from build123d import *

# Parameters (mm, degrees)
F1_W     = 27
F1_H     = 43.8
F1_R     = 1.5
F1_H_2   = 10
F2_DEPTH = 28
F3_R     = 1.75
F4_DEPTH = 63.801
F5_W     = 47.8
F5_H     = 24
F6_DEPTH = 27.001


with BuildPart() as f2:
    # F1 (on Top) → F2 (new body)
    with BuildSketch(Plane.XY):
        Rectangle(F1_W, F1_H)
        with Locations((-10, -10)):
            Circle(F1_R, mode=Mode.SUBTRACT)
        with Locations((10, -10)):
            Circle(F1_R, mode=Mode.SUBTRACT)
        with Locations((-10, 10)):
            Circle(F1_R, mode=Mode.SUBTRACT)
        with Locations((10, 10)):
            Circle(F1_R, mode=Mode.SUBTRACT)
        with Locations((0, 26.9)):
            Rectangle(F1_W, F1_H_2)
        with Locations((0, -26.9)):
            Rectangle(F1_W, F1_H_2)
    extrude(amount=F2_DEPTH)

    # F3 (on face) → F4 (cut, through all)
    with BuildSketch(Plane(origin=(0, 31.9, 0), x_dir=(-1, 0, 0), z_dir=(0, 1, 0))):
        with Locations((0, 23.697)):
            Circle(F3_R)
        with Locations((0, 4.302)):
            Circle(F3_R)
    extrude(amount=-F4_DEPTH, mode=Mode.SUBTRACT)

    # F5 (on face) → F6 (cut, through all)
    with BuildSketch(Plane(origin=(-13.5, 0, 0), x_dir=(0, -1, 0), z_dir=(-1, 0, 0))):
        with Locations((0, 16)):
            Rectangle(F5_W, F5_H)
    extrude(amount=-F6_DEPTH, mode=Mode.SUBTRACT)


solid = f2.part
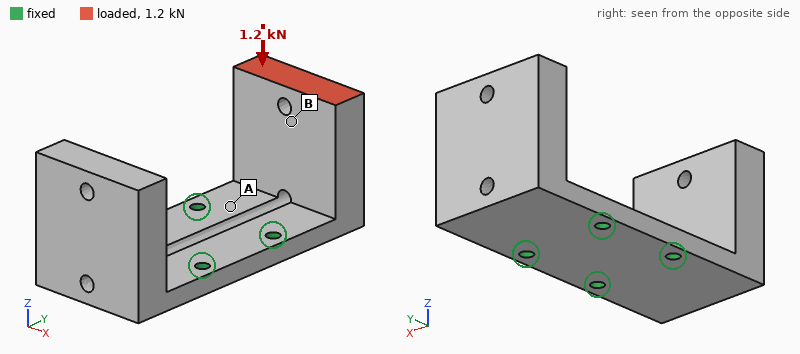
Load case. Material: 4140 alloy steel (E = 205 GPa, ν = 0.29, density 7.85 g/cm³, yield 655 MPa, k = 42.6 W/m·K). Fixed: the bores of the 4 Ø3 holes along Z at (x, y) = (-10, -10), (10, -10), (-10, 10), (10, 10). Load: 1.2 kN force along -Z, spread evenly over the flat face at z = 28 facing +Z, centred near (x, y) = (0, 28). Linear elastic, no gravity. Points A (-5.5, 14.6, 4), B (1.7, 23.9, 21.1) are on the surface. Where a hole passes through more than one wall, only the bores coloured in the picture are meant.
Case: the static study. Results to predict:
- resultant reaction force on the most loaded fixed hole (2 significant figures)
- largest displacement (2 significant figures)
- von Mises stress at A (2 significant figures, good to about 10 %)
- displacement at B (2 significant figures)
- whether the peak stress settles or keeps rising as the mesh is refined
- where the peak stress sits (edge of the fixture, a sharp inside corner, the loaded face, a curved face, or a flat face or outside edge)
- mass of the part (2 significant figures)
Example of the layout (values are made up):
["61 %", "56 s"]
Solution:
["720 N", "0.21 mm", "200 MPa", "0.14 mm", "keeps rising", "edge of the fixture", "130 g"]
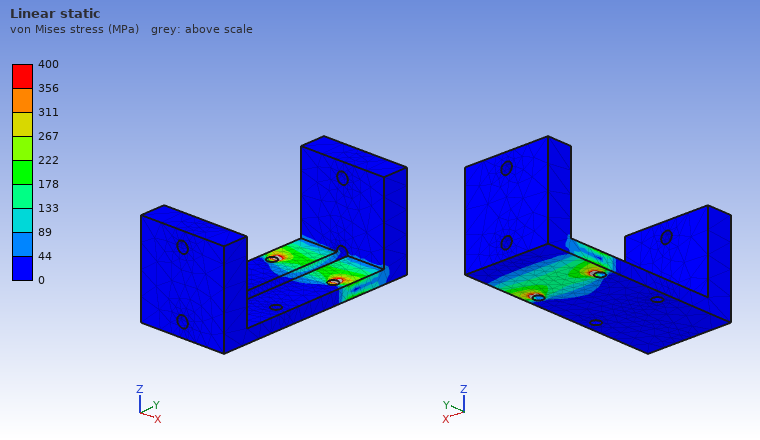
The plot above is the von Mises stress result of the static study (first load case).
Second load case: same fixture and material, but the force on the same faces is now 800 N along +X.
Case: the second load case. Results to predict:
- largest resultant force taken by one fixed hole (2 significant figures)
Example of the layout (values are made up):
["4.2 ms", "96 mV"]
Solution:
["1.3 kN"]
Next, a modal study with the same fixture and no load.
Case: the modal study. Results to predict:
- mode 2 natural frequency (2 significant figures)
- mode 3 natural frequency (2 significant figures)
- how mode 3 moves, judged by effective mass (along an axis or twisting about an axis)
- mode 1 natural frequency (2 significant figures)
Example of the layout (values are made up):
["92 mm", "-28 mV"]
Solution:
["1700 Hz", "3600 Hz", "along X", "1700 Hz"]
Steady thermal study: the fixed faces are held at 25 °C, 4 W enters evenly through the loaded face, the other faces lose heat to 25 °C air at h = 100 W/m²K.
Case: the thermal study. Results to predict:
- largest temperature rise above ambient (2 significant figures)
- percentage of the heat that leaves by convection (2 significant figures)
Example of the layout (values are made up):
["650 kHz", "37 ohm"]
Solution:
["15 K", "61 %"]
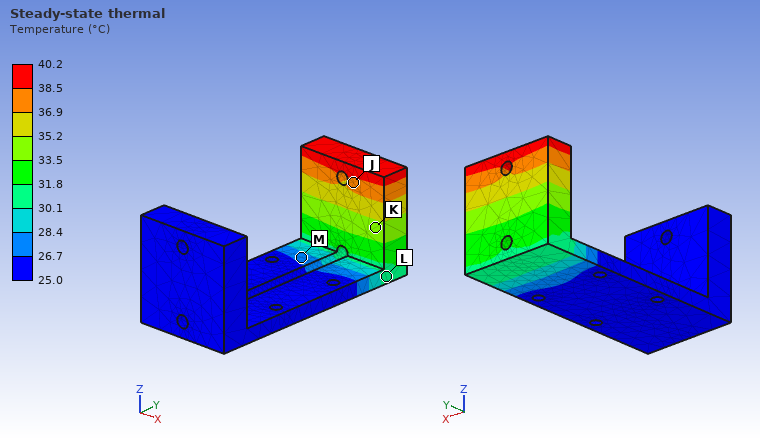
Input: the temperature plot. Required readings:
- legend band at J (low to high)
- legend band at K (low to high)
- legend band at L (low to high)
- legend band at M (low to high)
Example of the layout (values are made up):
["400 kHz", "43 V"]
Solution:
["36.9 to 38.5 °C", "33.5 to 35.2 °C", "30.1 to 31.8 °C", "26.7 to 28.4 °C"]
